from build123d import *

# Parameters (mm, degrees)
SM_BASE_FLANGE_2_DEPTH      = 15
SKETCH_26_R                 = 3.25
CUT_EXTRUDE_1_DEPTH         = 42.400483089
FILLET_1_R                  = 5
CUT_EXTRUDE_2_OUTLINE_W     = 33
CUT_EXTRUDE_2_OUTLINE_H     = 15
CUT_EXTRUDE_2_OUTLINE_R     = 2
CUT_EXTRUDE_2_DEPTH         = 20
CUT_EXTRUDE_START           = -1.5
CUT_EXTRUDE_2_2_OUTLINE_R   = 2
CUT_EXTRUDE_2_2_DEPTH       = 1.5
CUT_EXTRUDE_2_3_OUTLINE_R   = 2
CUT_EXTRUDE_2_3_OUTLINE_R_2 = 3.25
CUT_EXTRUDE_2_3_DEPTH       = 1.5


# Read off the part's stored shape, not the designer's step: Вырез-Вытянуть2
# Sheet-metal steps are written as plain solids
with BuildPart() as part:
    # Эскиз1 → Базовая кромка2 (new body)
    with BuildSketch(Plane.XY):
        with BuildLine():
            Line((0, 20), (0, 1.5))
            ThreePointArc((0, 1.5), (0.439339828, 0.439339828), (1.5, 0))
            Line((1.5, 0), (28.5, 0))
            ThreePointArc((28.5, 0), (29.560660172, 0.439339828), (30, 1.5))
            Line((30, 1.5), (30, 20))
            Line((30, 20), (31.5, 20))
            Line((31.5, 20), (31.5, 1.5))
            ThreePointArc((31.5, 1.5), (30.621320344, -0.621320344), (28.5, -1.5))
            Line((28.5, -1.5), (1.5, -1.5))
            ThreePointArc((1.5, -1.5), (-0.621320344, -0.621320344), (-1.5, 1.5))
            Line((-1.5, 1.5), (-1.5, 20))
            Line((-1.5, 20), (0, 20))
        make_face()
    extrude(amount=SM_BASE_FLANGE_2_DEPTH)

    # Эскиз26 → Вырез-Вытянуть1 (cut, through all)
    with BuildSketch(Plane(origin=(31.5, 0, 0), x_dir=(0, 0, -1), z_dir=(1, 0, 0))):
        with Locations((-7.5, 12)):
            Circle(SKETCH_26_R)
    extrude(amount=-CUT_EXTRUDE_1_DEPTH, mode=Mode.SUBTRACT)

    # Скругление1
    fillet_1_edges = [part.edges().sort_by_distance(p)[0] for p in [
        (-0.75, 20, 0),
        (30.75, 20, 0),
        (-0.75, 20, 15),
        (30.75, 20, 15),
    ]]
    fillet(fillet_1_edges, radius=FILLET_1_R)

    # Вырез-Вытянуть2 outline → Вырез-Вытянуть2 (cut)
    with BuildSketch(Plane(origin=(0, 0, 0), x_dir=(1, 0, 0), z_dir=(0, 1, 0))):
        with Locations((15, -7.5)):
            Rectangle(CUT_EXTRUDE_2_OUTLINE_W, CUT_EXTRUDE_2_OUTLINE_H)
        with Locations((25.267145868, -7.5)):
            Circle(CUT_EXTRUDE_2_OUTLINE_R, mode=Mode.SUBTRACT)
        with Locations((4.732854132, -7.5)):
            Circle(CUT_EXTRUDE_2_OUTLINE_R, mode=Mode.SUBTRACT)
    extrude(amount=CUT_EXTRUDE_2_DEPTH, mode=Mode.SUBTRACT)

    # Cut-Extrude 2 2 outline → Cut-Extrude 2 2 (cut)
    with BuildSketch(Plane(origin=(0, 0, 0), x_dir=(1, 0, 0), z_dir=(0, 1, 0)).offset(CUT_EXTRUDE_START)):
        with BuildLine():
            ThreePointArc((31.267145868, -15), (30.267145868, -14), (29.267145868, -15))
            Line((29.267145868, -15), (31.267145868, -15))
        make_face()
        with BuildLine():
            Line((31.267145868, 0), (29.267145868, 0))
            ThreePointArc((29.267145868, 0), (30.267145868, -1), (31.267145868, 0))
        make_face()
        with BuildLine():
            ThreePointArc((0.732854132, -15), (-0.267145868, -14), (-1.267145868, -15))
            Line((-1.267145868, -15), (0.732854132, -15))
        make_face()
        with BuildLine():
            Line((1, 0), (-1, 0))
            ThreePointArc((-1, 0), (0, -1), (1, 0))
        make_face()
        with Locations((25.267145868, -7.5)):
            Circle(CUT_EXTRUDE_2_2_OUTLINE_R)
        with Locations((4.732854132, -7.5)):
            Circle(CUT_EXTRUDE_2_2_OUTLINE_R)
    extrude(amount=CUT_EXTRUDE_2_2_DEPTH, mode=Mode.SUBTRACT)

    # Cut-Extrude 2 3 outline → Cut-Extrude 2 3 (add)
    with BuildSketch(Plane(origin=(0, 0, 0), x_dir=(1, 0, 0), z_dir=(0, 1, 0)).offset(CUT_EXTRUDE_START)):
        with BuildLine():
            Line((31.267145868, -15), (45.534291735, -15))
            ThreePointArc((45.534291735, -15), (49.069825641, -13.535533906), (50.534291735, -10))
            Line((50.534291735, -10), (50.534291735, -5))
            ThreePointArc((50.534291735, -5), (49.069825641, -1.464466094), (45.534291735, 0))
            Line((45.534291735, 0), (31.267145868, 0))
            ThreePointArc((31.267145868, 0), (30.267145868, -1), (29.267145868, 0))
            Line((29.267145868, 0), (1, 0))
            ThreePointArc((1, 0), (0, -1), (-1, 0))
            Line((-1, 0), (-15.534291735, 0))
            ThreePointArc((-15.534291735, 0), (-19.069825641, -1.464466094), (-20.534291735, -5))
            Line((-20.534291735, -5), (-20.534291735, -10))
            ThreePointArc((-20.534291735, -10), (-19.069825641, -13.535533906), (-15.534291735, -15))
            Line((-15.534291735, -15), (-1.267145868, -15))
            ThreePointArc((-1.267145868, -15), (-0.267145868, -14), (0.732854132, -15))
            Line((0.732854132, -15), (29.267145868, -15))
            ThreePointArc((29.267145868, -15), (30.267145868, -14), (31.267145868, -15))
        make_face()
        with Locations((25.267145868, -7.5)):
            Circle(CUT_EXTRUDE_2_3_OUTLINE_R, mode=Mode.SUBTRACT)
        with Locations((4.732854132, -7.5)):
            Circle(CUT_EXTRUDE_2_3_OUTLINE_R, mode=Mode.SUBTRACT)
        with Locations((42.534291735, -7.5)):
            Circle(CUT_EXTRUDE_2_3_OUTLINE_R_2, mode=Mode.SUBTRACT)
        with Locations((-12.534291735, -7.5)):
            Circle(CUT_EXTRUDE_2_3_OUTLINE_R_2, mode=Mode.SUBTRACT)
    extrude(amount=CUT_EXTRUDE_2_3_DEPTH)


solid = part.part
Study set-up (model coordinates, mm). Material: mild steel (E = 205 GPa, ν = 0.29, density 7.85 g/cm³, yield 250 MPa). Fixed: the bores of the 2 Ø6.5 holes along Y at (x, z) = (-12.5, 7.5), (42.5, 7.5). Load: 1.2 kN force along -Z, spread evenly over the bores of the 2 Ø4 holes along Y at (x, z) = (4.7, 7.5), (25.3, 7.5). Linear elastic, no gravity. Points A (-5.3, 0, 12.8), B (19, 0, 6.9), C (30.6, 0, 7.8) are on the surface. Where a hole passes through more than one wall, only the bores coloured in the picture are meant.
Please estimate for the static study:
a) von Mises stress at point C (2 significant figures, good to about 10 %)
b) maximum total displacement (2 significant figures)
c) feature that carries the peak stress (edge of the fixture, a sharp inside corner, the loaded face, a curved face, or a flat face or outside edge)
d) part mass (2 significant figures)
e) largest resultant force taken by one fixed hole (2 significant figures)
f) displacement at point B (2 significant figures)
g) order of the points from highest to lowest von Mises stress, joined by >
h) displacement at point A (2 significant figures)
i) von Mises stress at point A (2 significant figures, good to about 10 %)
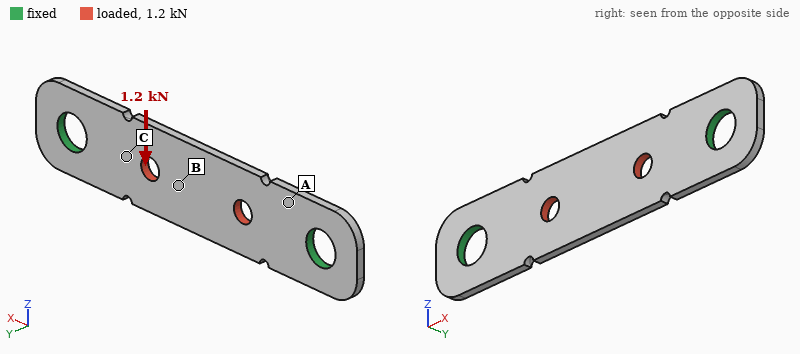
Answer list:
77 MPa
17 µm
edge of the fixture
11 g
600 N
17 µm
C > A > B
5.2 µm
43 MPa
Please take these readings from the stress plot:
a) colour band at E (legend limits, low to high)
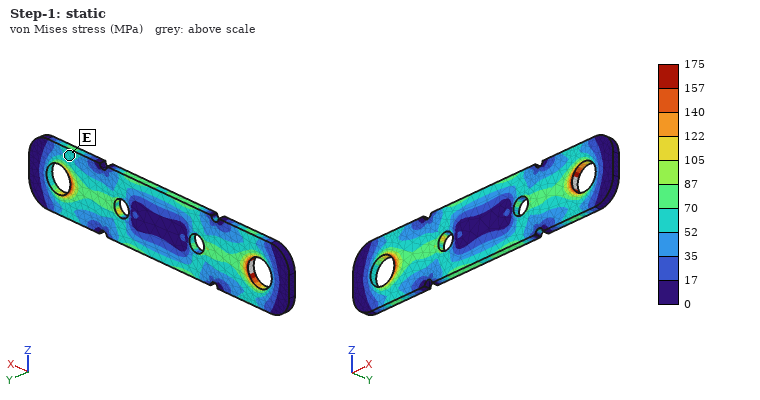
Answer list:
52 to 70 MPa
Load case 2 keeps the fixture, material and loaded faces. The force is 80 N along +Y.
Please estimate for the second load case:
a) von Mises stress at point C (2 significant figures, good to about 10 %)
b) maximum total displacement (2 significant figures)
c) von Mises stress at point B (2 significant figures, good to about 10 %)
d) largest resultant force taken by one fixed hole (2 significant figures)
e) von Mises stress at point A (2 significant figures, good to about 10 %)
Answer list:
9.7 MPa
39 µm
24 MPa
40 N
39 MPa
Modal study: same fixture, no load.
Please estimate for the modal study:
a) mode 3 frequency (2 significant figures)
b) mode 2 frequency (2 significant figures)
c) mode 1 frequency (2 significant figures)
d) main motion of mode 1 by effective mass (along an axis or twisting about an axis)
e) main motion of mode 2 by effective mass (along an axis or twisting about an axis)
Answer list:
8400 Hz
6400 Hz
3200 Hz
along Y
twisting about X
